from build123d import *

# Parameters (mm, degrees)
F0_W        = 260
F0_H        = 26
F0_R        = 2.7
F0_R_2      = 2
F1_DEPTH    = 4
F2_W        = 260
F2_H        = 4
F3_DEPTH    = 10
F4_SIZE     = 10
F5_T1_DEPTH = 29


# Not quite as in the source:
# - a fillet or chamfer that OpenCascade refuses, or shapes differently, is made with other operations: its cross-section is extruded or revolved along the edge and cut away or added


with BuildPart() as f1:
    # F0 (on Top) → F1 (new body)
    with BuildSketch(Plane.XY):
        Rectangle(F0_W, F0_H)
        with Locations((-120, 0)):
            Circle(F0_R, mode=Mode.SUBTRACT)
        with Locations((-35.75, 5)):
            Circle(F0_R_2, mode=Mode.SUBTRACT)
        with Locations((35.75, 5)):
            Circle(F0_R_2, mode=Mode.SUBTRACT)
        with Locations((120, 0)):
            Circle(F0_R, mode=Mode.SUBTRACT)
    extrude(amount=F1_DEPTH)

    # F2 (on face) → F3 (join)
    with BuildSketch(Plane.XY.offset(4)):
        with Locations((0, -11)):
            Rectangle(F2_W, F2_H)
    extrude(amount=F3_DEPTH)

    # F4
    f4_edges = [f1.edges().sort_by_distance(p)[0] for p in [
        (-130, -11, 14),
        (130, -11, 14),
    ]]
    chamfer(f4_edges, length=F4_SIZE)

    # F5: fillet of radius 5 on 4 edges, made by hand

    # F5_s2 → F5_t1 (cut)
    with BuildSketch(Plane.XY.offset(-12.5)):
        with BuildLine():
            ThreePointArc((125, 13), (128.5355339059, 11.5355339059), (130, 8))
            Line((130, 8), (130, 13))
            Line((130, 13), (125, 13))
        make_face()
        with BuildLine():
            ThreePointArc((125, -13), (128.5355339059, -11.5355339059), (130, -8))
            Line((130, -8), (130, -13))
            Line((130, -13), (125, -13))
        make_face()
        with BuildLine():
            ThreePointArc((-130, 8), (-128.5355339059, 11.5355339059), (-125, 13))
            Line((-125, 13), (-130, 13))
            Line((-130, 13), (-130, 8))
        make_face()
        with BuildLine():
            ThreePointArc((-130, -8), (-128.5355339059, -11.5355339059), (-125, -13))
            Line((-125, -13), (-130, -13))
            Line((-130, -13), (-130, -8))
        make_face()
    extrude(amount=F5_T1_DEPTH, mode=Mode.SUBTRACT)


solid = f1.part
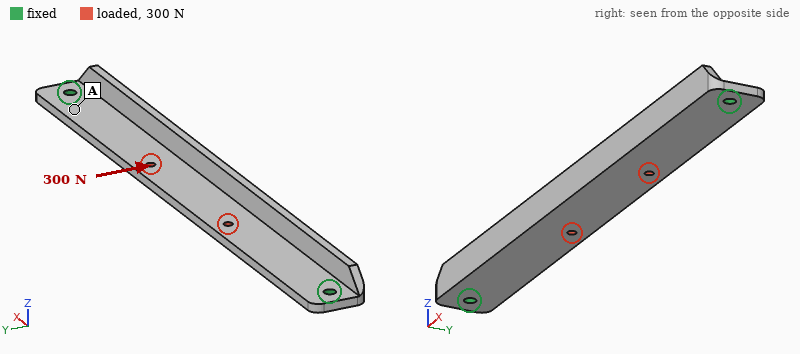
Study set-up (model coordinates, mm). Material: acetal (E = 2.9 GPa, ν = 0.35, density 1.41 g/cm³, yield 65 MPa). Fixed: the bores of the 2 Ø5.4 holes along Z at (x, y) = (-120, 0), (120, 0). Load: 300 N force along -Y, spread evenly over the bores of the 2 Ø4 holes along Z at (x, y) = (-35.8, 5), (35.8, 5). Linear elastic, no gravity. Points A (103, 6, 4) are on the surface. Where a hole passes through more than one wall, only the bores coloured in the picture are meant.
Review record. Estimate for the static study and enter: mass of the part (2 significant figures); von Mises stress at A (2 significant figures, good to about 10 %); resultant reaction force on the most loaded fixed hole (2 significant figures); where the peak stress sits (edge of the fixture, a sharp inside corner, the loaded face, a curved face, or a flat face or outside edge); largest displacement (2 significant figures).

52 g
7.4 MPa
170 N
edge of the fixture
2.3 mm
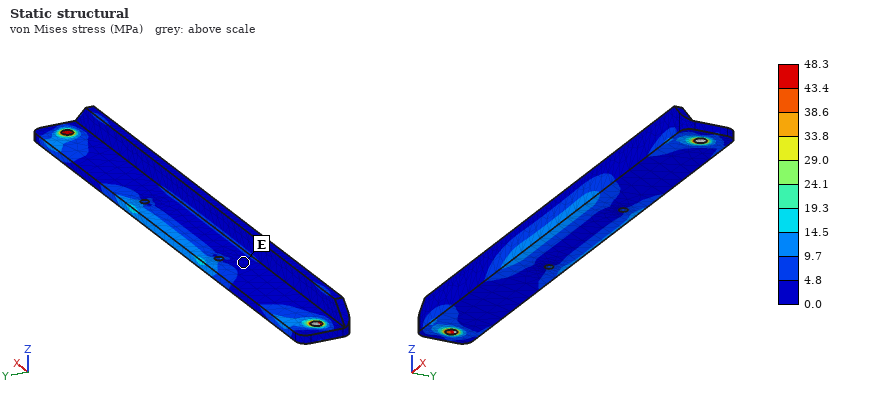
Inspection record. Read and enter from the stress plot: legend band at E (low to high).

0.0 to 4.8 MPa
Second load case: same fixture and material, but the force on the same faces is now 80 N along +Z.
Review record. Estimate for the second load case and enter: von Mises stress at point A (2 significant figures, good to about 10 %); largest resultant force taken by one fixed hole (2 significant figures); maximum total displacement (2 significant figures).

5.1 MPa
87 N
3.1 mm
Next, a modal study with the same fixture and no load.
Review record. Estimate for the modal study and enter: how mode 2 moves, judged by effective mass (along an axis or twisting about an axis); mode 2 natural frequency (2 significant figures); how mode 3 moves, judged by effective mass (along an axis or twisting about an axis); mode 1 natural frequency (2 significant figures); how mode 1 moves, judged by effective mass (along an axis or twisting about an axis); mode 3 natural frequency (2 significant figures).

along Y
390 Hz
twisting about Y
190 Hz
along Z
530 Hz
